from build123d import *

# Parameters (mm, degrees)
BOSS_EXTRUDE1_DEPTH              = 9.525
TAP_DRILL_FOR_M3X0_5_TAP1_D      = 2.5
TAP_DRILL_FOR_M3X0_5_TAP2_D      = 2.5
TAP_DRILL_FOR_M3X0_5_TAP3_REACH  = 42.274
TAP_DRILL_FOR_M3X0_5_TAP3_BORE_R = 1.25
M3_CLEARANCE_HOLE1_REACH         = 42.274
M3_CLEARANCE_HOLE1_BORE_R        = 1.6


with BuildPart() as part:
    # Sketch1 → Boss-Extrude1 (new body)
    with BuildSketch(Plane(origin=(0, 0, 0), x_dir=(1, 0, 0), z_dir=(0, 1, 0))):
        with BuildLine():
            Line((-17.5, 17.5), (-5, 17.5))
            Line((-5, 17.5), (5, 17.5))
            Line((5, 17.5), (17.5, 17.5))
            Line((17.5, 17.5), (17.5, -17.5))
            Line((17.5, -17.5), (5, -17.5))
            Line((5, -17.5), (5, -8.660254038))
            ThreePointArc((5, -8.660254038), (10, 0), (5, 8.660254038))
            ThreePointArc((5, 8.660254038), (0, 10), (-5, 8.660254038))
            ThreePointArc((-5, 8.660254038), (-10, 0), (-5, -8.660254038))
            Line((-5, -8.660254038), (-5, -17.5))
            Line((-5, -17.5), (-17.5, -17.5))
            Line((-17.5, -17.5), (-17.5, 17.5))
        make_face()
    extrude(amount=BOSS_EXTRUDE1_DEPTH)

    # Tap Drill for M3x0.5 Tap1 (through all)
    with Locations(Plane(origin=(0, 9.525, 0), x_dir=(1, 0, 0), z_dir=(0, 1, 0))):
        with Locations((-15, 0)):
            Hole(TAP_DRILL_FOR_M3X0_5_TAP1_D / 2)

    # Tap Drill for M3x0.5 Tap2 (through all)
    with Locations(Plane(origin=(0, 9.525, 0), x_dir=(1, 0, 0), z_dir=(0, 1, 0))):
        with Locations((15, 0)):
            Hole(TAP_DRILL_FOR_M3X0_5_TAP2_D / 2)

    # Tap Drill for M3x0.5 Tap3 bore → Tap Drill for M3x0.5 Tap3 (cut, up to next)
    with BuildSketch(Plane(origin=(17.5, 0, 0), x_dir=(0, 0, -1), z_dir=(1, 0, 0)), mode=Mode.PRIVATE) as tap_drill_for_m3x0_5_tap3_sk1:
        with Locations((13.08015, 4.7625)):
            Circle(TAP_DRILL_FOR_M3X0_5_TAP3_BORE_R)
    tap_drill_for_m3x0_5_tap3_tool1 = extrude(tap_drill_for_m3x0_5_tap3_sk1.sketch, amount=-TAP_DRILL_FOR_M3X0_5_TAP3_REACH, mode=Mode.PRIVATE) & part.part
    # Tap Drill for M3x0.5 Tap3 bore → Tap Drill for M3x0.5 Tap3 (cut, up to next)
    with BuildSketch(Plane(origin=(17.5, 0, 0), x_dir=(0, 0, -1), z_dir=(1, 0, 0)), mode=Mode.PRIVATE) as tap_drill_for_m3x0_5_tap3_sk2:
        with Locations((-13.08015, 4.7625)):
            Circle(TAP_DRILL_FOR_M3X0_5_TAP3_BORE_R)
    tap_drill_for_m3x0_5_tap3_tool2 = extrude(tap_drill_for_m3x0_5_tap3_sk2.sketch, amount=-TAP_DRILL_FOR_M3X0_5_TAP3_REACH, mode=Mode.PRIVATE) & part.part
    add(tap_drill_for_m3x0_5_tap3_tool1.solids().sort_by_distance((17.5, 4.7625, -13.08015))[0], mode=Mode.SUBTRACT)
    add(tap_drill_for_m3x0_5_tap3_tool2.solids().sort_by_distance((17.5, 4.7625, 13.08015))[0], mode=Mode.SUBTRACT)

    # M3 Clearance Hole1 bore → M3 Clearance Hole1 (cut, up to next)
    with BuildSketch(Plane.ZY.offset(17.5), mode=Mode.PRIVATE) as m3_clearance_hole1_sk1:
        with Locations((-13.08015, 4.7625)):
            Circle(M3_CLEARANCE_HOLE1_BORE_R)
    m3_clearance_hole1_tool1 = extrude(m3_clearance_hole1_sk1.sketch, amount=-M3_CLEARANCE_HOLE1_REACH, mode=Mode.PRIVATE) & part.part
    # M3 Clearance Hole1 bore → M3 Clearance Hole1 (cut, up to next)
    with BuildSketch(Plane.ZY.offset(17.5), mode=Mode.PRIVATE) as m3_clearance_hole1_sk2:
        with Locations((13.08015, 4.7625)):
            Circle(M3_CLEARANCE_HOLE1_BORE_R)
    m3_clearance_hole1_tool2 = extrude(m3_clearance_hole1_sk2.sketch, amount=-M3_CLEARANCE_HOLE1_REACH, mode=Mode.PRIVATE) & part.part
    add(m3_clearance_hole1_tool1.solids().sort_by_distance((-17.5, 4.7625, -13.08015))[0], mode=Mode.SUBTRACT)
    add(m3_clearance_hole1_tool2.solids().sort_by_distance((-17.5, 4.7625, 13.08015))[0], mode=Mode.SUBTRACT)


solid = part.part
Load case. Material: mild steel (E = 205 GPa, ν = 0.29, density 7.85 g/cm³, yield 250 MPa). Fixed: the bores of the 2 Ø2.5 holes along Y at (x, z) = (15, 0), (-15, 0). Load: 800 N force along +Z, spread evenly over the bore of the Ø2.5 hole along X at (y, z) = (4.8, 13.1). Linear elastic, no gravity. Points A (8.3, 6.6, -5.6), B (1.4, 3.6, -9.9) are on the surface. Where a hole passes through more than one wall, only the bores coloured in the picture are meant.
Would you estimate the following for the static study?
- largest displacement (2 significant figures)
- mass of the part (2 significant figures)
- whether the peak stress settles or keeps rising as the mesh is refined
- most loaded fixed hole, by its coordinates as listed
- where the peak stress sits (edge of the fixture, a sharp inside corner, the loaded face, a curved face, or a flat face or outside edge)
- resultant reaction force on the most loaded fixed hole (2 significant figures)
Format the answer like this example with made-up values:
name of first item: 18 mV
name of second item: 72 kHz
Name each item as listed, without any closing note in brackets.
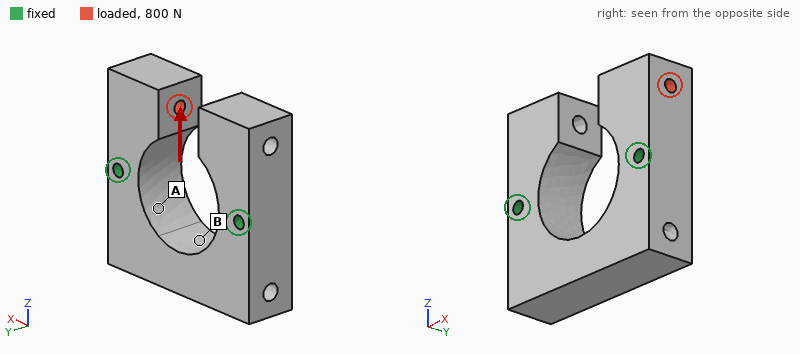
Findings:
largest displacement: 5.5 µm
mass of the part: 58 g
whether the peak stress settles or keeps rising as the mesh is refined: keeps rising
most loaded fixed hole, by its coordinates as listed: (15, 0)
where the peak stress sits: edge of the fixture
resultant reaction force on the most loaded fixed hole: 760 N
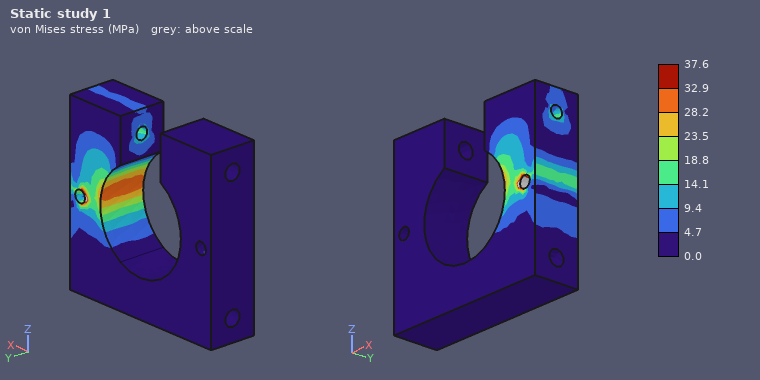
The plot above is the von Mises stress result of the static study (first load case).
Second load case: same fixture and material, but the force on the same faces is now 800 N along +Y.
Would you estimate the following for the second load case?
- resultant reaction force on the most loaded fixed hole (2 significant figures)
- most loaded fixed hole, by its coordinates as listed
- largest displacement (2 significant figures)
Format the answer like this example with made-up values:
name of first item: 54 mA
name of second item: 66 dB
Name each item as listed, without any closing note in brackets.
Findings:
resultant reaction force on the most loaded fixed hole: 810 N
most loaded fixed hole, by its coordinates as listed: (15, 0)
largest displacement: 12 µm
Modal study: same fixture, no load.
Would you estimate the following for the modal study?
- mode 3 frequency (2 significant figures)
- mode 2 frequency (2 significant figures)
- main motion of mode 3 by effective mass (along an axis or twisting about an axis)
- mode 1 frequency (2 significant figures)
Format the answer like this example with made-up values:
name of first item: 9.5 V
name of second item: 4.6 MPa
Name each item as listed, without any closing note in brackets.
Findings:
mode 3 frequency: 14 kHz
mode 2 frequency: 13 kHz
main motion of mode 3 by effective mass: along Y
mode 1 frequency: 12 kHz
